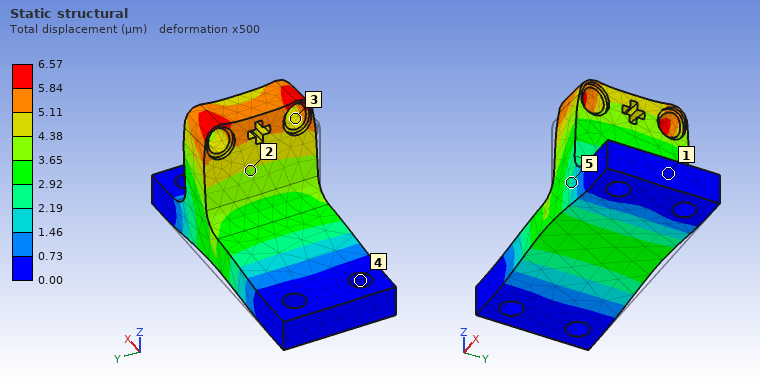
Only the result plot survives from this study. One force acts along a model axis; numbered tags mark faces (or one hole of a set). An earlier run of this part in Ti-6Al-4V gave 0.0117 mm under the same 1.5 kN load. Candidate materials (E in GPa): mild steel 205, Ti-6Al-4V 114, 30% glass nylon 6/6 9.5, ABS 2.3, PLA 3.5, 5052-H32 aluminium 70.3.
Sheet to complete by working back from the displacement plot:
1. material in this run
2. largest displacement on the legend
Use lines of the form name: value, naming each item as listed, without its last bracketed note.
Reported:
material in this run: mild steel
largest displacement on the legend: 6.57 µm
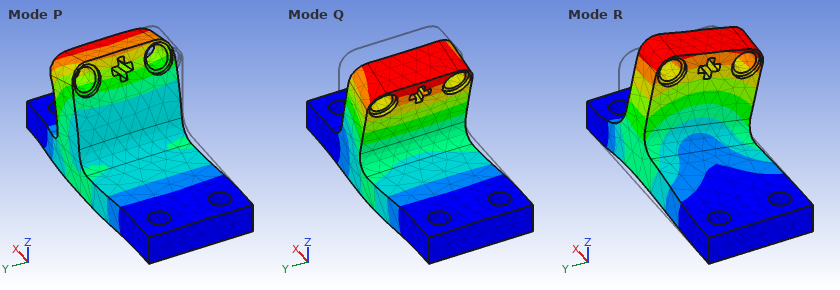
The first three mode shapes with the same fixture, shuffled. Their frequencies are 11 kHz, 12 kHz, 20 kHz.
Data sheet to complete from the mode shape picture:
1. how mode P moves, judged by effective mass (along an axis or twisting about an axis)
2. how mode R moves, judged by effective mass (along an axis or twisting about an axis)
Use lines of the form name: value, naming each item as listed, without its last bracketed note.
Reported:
how mode P moves, judged by effective mass: along Z
how mode R moves, judged by effective mass: along Y
